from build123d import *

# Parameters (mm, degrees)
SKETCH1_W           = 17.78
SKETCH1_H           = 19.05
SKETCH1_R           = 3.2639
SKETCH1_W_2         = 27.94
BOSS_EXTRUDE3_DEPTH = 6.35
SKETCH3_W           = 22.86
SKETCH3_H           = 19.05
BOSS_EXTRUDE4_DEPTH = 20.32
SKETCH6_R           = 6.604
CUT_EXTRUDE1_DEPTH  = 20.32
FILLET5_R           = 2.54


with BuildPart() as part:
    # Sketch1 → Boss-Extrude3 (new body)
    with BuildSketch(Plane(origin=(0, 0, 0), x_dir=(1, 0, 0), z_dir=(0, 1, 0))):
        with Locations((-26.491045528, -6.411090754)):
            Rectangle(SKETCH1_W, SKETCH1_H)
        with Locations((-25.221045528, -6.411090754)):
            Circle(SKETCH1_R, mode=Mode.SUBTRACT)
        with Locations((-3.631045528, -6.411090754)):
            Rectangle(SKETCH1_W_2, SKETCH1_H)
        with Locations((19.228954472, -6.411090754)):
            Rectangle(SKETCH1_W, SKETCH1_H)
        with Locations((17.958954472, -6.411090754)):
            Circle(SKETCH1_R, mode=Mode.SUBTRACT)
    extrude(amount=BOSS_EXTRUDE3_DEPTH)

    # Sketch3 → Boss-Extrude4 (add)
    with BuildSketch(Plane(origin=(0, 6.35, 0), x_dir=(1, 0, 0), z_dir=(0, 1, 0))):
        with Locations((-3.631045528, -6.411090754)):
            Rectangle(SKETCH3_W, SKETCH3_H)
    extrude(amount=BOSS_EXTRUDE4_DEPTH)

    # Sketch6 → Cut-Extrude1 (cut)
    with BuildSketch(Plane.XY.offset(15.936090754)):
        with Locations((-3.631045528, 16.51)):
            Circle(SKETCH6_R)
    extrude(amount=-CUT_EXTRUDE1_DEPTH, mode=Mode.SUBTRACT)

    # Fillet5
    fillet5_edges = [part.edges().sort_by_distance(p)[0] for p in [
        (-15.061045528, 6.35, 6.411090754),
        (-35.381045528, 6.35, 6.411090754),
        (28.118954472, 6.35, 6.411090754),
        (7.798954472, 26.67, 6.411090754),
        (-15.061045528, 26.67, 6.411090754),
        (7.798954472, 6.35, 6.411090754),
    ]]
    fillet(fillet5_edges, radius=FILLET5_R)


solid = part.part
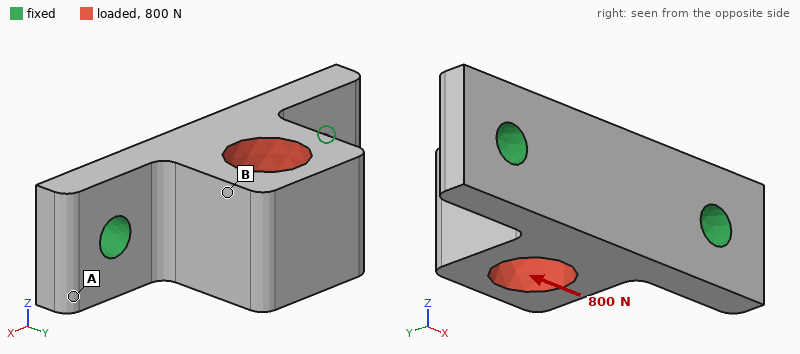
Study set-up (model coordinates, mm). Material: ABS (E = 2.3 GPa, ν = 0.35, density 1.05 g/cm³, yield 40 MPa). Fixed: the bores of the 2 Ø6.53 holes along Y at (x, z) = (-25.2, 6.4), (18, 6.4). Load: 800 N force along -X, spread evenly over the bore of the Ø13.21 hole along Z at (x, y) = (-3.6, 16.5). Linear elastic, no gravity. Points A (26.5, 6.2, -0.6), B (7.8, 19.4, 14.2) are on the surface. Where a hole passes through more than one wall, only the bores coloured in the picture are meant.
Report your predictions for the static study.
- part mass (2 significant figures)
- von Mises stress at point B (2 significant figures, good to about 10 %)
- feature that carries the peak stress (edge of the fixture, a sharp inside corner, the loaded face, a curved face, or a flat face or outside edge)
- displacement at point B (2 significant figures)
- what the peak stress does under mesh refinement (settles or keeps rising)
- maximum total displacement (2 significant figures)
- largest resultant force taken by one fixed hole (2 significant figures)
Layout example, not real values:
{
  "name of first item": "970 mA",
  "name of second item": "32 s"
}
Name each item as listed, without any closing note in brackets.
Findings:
{
  "part mass": "14 g",
  "von Mises stress at point B": "4.0 MPa",
  "feature that carries the peak stress": "edge of the fixture",
  "displacement at point B": "0.19 mm",
  "what the peak stress does under mesh refinement": "keeps rising",
  "maximum total displacement": "0.25 mm",
  "largest resultant force taken by one fixed hole": "510 N"
}
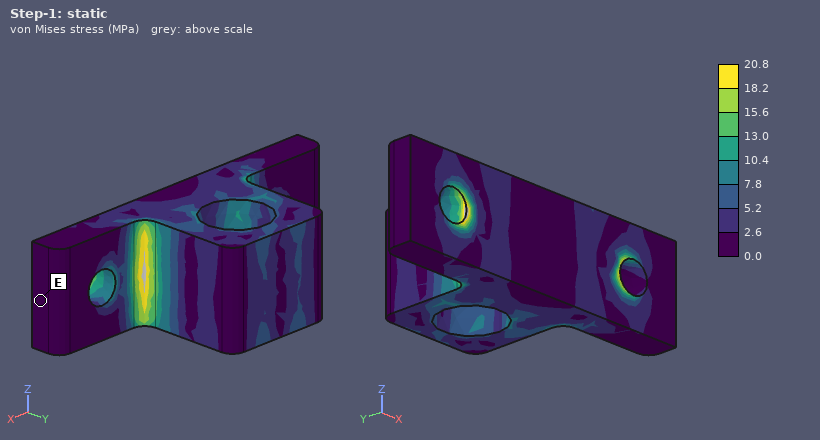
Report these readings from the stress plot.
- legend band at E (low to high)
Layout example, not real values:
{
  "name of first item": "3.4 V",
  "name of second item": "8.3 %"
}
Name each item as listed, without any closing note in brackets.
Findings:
{
  "legend band at E": "0.0 to 2.6 MPa"
}
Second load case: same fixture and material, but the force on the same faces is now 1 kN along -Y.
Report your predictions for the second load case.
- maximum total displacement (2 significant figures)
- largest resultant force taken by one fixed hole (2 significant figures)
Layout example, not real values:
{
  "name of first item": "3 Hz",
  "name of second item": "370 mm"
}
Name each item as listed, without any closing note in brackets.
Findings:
{
  "maximum total displacement": "0.16 mm",
  "largest resultant force taken by one fixed hole": "550 N"
}
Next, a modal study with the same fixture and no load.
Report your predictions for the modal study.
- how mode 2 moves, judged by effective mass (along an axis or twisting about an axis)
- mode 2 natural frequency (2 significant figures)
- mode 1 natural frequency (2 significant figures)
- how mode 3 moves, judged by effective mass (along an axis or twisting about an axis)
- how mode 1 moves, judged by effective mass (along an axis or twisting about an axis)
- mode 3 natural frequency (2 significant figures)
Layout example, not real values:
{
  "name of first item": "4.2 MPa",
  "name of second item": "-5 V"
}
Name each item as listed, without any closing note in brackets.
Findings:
{
  "how mode 2 moves, judged by effective mass": "along X",
  "mode 2 natural frequency": "3900 Hz",
  "mode 1 natural frequency": "1900 Hz",
  "how mode 3 moves, judged by effective mass": "along Y",
  "how mode 1 moves, judged by effective mass": "along Z",
  "mode 3 natural frequency": "4300 Hz"
}
